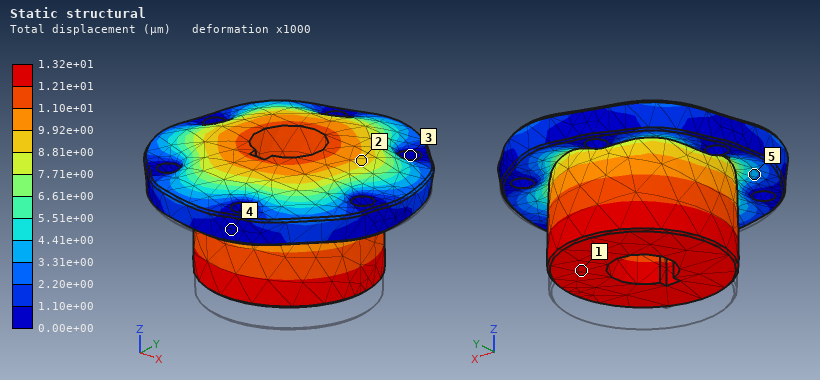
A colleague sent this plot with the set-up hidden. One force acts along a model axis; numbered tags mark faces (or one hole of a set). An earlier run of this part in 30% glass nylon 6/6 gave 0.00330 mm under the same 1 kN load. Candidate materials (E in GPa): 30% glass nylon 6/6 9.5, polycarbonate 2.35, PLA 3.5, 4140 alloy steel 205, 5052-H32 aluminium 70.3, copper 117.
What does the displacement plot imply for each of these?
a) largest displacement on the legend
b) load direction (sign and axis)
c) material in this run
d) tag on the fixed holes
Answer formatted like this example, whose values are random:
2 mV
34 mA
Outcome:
1.32e+01 µm
+Z
polycarbonate
3
